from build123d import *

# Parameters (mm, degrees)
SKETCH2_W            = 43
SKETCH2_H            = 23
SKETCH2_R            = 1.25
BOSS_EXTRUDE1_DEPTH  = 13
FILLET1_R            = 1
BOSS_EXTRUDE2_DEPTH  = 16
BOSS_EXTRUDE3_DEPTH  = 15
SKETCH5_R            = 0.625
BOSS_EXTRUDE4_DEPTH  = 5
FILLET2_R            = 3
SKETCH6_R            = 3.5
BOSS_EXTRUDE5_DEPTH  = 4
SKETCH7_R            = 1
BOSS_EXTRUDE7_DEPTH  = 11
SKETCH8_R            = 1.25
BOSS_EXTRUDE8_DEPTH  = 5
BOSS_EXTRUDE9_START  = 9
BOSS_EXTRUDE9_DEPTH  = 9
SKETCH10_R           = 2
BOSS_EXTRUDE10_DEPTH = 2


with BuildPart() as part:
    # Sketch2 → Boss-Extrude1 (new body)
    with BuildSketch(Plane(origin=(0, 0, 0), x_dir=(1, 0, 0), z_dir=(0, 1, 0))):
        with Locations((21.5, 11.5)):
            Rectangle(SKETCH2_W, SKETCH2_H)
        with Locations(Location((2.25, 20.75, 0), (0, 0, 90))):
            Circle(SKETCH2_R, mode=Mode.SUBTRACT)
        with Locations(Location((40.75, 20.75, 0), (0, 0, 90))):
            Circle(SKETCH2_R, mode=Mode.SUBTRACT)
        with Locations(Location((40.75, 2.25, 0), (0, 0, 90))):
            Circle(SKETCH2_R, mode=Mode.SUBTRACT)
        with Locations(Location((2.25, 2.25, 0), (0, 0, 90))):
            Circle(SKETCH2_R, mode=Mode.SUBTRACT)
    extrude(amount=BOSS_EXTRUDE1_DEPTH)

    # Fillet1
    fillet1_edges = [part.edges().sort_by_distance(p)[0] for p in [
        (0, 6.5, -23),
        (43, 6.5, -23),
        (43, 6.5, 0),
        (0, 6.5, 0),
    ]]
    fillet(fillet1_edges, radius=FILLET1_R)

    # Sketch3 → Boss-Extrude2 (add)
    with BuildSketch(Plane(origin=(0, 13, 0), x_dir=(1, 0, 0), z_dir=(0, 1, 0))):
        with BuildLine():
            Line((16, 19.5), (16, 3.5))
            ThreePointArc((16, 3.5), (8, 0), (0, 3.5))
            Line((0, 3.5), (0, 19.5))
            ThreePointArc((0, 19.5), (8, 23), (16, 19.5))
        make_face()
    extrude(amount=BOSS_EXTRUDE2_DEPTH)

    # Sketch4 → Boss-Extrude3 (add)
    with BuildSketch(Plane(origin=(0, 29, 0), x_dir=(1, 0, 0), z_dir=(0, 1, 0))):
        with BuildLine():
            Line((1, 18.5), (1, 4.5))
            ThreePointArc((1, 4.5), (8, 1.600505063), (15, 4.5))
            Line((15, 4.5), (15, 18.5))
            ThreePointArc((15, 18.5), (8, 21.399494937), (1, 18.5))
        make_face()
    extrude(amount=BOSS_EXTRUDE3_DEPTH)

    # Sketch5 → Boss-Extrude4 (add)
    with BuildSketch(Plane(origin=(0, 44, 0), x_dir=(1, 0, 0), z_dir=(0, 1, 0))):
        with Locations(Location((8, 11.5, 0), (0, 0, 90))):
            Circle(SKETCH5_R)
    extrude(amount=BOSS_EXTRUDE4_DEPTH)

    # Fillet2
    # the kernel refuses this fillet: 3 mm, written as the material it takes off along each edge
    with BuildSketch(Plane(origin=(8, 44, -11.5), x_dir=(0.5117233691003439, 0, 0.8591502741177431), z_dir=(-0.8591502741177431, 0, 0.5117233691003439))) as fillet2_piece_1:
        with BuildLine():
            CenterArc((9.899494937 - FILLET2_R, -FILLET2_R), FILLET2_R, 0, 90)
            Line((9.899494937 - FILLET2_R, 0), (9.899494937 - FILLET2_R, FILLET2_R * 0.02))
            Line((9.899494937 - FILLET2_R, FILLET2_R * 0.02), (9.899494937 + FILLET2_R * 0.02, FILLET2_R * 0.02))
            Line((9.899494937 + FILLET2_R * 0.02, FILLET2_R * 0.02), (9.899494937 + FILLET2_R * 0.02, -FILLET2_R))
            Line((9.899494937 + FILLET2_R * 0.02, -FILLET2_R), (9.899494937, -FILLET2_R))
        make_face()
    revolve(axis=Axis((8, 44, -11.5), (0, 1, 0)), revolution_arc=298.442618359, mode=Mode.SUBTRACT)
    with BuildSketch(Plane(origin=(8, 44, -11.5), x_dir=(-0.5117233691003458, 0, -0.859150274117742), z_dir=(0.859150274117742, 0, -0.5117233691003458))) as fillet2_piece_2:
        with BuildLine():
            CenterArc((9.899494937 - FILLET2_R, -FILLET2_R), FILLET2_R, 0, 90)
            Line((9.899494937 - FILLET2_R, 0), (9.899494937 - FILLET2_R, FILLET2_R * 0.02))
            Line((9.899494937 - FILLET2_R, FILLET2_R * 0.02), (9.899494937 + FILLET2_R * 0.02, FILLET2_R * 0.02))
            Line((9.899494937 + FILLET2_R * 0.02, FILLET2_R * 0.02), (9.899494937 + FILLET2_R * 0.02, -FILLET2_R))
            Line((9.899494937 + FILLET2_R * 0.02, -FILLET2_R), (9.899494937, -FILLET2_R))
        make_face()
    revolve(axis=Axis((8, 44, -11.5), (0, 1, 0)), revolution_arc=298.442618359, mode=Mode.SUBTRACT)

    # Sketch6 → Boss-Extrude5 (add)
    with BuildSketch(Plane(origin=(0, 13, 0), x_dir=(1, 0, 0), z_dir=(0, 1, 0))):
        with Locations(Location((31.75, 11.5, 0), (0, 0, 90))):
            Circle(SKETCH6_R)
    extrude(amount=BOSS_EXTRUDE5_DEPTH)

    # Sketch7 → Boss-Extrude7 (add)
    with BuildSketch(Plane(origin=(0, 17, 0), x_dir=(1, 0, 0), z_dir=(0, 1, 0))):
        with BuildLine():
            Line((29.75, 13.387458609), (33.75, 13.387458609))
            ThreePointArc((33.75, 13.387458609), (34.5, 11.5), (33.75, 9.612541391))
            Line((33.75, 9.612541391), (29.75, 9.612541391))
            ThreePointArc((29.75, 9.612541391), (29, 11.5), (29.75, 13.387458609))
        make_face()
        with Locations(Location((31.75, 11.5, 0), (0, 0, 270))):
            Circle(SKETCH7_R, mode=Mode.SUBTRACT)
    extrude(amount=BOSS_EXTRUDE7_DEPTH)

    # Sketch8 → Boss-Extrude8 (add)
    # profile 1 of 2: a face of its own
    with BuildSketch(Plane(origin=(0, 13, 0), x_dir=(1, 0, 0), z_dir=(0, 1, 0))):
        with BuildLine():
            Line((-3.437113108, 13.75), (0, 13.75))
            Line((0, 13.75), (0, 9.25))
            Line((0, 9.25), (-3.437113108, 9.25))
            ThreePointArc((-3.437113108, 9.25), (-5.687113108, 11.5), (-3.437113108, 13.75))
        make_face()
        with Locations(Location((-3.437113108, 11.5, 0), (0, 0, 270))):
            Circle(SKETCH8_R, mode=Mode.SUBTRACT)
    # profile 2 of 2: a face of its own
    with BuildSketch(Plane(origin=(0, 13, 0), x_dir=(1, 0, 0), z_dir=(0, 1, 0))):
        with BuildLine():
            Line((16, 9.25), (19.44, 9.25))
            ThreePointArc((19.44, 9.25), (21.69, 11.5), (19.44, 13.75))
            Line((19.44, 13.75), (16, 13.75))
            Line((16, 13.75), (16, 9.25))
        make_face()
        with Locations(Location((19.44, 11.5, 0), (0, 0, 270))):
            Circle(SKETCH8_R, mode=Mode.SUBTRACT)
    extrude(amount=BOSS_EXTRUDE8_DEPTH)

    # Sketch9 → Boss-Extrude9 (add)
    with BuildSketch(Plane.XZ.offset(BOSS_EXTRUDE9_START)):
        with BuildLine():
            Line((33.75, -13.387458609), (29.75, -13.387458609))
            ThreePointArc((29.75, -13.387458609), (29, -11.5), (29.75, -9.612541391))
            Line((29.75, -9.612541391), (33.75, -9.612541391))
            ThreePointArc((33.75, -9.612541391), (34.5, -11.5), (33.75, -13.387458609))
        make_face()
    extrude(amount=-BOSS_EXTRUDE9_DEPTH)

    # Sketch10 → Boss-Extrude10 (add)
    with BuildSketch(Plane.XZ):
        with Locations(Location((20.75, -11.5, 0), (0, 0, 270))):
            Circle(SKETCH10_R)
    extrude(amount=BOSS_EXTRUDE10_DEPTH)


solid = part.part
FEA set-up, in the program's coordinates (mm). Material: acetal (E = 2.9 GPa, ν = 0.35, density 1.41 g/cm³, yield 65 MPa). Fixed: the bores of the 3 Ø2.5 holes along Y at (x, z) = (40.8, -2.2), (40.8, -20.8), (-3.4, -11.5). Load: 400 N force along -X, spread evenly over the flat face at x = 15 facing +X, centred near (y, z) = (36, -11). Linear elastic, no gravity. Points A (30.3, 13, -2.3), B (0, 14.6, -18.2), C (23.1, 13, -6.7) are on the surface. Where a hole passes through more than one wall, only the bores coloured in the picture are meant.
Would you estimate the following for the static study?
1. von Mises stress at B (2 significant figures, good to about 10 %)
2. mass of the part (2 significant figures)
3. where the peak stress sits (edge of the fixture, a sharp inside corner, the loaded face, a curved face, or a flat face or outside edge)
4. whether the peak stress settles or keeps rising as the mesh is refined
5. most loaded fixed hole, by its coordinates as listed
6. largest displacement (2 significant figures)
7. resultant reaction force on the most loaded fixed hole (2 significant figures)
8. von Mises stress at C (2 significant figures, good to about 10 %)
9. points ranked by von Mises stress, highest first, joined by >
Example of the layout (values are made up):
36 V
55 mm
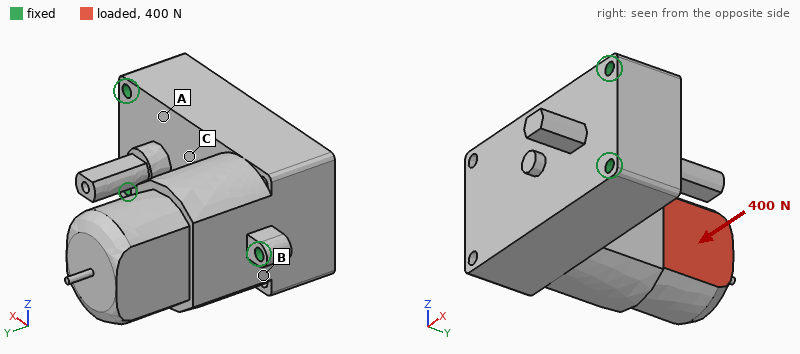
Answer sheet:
6.3 MPa
32 g
edge of the fixture
keeps rising
(-3.4, -11.5)
0.34 mm
470 N
3.5 MPa
B > C > A
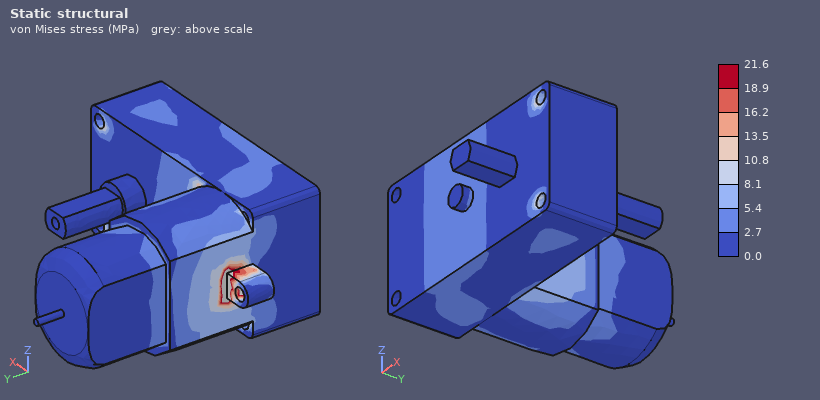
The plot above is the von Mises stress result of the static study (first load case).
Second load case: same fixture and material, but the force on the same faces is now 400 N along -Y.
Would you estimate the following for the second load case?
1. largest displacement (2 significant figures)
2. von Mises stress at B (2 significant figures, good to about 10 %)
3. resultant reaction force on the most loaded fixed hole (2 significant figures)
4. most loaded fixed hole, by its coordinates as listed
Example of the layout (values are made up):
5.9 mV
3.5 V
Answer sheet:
0.16 mm
2.9 MPa
200 N
(-3.4, -11.5)
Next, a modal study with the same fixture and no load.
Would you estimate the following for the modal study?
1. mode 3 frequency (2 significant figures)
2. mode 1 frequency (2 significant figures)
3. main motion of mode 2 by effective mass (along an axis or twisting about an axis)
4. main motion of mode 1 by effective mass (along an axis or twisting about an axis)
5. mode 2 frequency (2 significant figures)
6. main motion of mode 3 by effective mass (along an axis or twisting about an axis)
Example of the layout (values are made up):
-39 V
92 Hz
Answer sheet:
2900 Hz
1500 Hz
along X
along Z
2600 Hz
along Y
